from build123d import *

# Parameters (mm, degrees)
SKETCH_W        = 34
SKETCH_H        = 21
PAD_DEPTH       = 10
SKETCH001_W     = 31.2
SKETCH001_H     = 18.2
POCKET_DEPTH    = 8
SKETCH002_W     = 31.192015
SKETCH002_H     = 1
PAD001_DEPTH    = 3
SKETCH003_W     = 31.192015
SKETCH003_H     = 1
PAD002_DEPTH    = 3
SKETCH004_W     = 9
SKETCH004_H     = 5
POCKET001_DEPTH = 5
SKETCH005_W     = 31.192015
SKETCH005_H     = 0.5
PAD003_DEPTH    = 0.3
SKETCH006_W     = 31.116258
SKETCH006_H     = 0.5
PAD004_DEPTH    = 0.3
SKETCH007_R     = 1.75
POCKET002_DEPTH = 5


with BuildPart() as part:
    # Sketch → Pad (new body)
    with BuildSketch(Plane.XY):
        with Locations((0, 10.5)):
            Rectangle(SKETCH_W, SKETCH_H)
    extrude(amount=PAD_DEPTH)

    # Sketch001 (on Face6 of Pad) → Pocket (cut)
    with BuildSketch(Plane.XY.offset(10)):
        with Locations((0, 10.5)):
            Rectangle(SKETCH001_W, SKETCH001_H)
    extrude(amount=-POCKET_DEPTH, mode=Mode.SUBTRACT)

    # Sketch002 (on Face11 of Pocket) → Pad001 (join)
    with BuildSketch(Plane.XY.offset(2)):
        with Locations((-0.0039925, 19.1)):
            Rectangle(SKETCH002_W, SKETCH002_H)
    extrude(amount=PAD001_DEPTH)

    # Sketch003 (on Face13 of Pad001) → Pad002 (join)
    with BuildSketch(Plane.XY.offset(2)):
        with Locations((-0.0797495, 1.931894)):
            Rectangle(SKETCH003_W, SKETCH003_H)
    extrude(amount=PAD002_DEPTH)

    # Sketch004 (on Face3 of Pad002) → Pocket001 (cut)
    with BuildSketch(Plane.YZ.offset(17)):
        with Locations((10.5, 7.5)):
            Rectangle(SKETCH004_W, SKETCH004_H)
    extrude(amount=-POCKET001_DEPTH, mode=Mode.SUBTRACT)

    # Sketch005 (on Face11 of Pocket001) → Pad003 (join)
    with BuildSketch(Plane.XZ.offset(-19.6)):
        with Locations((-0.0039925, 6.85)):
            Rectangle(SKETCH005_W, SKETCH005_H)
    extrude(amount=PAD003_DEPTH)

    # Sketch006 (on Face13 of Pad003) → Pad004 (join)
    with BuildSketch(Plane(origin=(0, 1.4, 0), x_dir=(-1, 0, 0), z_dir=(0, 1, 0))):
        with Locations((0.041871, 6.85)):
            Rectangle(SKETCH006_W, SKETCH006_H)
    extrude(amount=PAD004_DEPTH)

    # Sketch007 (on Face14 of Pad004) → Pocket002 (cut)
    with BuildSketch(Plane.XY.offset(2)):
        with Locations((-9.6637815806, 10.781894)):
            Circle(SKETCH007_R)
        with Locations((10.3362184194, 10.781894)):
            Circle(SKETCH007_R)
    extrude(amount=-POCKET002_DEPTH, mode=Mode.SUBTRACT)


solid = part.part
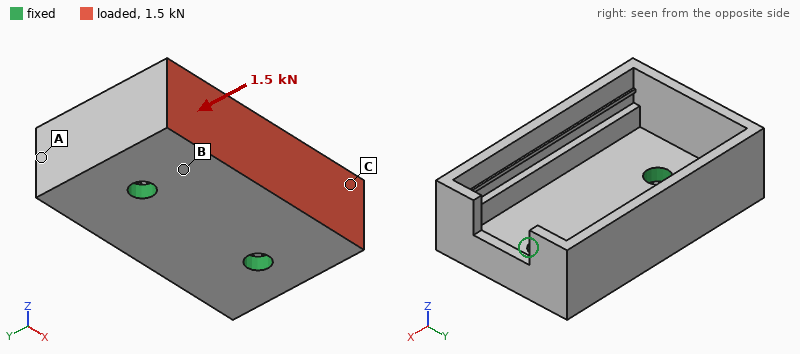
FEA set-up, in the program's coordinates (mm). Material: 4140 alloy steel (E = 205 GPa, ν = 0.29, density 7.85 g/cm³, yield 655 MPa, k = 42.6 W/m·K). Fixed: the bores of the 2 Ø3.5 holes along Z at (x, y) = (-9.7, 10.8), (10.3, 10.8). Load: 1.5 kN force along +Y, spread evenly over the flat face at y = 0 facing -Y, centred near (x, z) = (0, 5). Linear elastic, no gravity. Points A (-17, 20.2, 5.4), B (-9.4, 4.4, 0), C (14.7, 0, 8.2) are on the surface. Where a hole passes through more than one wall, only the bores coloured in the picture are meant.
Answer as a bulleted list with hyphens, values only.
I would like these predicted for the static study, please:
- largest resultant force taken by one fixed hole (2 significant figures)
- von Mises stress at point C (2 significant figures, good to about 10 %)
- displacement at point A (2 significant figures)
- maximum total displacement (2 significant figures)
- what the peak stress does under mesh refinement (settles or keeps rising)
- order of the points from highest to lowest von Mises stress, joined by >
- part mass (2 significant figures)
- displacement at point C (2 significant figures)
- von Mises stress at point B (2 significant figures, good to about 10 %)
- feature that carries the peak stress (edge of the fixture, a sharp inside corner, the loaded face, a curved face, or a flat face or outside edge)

- 800 N
- 140 MPa
- 0.024 mm
- 0.11 mm
- keeps rising
- C > B > A
- 21 g
- 0.052 mm
- 78 MPa
- edge of the fixture
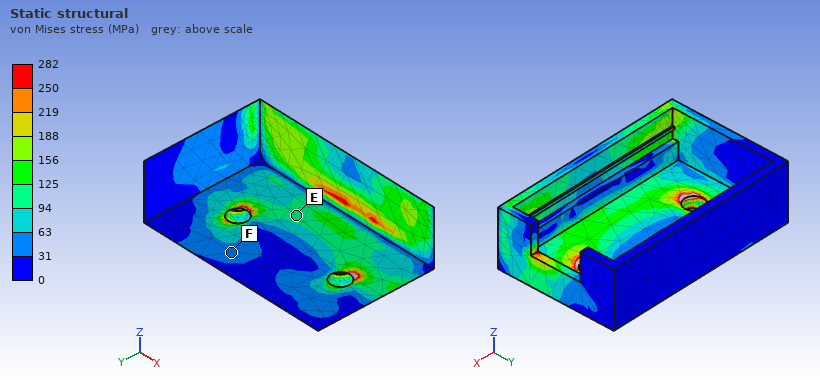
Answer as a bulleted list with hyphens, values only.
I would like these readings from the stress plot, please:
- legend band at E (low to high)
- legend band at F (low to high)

- 94 to 125 MPa
- 31 to 63 MPa
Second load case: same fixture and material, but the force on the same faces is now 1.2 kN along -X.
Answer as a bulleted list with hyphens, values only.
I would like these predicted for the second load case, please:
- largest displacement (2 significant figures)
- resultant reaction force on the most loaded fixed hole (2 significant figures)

- 29 µm
- 860 N
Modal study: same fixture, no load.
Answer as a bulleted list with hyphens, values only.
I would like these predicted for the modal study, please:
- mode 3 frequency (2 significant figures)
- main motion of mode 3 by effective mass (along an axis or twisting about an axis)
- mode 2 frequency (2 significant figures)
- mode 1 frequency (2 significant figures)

- 12 kHz
- along Z
- 9000 Hz
- 7200 Hz
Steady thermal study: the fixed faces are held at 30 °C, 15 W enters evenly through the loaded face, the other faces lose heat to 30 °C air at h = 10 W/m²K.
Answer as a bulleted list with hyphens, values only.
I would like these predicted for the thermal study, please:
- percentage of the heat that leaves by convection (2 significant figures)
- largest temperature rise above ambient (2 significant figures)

- 4.9 %
- 72 K
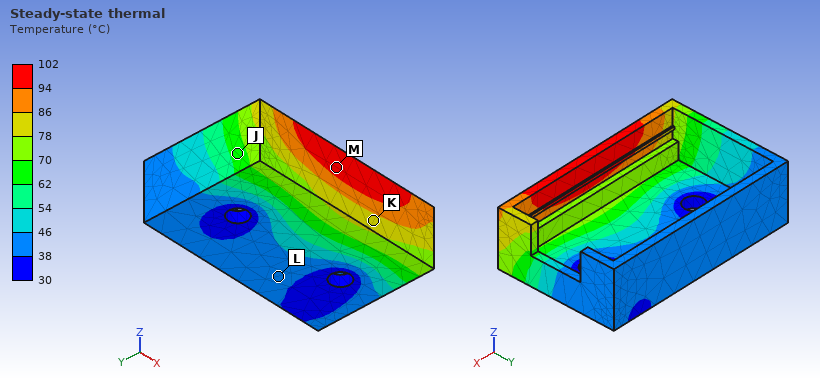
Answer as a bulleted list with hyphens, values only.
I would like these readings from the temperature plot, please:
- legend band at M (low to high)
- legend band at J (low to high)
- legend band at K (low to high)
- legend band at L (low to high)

- 94 to 102 °C
- 62 to 70 °C
- 78 to 86 °C
- 38 to 46 °C
